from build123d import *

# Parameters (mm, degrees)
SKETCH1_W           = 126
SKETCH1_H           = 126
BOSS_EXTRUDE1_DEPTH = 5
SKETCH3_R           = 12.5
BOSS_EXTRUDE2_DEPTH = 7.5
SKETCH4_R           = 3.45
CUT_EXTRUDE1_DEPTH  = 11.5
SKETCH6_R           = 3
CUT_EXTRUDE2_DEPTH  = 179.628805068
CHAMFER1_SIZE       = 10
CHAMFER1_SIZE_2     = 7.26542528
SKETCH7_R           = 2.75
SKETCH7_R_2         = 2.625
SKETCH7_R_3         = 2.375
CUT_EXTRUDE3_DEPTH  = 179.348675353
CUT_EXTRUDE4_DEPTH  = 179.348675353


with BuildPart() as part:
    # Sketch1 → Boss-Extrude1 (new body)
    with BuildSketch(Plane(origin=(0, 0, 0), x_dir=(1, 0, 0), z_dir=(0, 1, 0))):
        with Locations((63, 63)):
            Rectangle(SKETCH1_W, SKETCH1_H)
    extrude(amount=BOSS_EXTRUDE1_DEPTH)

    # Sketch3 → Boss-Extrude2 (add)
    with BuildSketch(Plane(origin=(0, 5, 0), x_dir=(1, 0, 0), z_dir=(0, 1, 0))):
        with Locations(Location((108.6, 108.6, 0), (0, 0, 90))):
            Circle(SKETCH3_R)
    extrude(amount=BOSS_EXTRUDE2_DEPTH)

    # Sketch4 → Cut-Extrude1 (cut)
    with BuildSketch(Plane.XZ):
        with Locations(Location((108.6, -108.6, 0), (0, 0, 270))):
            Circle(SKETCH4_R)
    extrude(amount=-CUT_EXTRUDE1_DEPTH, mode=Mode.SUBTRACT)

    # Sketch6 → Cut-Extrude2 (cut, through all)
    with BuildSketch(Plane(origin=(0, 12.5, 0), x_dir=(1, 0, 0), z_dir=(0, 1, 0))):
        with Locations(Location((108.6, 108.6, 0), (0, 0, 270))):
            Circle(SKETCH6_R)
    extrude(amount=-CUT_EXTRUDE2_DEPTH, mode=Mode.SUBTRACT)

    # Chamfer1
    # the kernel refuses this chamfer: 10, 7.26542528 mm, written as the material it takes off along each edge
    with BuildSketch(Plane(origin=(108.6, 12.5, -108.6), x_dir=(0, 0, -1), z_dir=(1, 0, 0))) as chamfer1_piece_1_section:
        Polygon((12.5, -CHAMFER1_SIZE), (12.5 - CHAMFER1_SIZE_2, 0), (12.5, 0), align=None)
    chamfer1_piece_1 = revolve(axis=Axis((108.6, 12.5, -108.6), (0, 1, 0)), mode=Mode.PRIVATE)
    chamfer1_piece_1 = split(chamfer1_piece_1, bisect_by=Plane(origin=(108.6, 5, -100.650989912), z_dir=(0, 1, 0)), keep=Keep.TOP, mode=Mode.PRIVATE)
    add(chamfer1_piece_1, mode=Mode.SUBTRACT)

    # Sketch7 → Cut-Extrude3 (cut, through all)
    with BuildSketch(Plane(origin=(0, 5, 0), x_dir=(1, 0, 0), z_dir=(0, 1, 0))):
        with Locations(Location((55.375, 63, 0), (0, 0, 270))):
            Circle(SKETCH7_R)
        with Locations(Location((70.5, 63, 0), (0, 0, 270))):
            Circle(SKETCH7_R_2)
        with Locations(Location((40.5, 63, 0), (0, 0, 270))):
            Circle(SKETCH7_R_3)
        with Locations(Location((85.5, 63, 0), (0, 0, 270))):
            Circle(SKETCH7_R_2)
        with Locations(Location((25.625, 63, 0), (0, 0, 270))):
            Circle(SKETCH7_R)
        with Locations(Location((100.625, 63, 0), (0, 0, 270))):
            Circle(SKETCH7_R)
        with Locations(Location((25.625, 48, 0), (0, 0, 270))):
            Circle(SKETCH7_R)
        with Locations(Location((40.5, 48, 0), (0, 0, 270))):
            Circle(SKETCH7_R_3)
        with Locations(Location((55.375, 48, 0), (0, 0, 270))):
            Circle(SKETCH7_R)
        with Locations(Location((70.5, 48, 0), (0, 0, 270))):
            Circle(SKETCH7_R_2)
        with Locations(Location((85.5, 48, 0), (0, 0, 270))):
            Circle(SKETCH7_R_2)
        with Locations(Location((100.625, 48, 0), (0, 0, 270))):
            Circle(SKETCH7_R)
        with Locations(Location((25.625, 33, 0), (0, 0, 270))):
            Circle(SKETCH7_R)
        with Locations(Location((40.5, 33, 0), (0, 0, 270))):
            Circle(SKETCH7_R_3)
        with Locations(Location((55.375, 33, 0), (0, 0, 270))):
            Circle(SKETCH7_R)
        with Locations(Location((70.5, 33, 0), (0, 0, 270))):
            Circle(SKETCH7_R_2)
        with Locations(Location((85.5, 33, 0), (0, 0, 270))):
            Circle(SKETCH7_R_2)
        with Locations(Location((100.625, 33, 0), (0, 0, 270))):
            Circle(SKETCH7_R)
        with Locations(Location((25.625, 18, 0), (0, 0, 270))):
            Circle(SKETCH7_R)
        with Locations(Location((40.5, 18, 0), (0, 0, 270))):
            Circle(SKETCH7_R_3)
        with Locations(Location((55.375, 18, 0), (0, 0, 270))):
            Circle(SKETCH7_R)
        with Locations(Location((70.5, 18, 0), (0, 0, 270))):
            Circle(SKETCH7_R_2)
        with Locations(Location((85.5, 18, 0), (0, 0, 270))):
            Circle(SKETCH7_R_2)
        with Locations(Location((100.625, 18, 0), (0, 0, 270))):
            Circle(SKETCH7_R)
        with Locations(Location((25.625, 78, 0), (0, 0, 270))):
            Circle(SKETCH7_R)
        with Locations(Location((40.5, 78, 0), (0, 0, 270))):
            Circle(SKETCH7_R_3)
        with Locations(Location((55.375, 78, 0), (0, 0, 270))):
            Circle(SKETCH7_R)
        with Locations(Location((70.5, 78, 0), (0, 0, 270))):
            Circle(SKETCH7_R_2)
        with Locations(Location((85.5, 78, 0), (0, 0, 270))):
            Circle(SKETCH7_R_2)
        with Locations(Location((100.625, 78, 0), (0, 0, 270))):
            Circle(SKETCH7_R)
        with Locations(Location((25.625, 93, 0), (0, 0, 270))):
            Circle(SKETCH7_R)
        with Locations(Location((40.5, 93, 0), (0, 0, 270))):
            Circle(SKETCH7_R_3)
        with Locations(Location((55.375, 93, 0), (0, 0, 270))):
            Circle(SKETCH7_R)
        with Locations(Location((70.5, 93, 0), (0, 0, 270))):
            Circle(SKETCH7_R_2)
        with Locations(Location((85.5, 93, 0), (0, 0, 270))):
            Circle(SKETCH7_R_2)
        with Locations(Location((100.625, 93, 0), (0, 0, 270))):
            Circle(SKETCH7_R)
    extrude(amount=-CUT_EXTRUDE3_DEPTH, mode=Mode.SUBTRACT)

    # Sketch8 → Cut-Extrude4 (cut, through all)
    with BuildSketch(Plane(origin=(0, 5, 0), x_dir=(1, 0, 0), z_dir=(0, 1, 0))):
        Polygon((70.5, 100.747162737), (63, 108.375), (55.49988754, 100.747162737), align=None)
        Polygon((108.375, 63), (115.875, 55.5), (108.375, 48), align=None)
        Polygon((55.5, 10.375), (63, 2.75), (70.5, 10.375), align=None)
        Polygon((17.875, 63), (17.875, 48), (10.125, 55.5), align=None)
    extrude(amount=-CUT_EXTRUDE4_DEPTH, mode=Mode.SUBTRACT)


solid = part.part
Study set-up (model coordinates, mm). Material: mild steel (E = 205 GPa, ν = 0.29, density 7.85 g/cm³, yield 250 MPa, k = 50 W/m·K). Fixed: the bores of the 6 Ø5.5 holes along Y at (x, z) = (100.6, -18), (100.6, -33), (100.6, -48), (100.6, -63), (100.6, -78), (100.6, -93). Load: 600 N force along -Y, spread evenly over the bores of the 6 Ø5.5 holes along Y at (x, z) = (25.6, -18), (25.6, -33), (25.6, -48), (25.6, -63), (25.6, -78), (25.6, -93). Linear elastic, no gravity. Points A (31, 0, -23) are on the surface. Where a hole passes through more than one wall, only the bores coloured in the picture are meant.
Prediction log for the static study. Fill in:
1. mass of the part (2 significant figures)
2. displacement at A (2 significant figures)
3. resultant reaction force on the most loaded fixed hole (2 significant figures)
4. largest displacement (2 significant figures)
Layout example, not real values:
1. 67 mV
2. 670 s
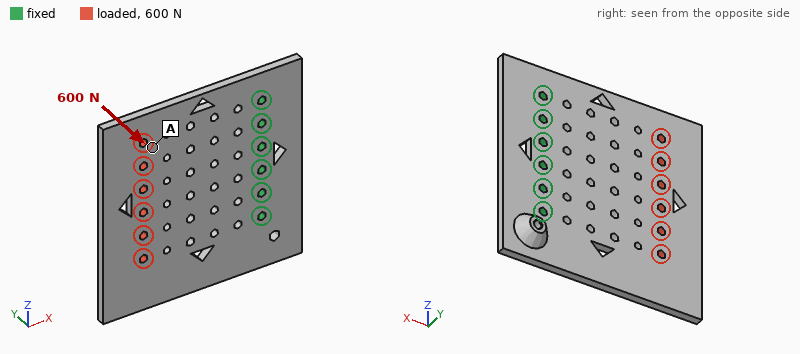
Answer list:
1. 590 g
2. 0.31 mm
3. 140 N
4. 0.54 mm
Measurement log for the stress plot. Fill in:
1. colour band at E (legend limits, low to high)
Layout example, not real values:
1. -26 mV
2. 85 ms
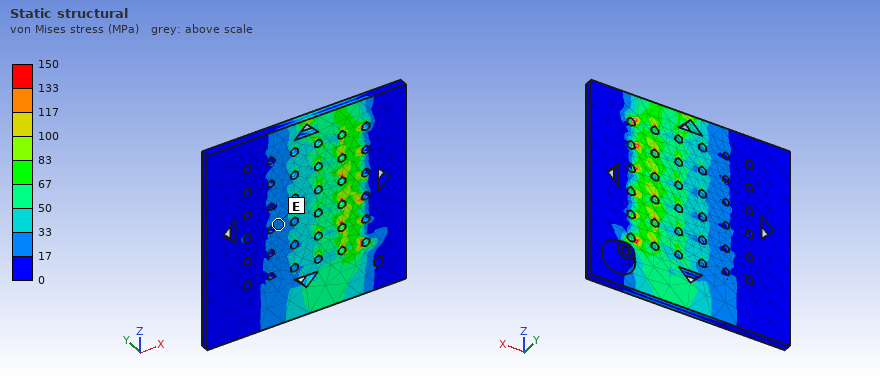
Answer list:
1. 17 to 33 MPa
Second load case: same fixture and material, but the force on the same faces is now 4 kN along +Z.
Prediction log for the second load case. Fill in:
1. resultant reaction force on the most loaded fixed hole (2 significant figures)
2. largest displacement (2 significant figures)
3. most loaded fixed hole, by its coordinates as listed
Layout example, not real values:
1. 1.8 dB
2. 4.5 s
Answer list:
1. 3.7 kN
2. 24 µm
3. (100.6, -93)
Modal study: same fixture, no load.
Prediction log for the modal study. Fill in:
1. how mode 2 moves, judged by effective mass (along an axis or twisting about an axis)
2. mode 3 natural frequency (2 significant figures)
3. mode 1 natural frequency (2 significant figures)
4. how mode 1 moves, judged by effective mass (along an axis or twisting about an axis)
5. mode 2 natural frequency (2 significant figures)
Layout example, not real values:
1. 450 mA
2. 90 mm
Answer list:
1. twisting about X
2. 2000 Hz
3. 400 Hz
4. along Y
5. 790 Hz
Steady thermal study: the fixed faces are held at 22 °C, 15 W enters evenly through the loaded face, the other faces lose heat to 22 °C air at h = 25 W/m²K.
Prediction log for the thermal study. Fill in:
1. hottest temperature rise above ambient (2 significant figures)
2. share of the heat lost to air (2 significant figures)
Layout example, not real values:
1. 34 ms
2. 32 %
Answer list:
1. 26 K
2. 60 %
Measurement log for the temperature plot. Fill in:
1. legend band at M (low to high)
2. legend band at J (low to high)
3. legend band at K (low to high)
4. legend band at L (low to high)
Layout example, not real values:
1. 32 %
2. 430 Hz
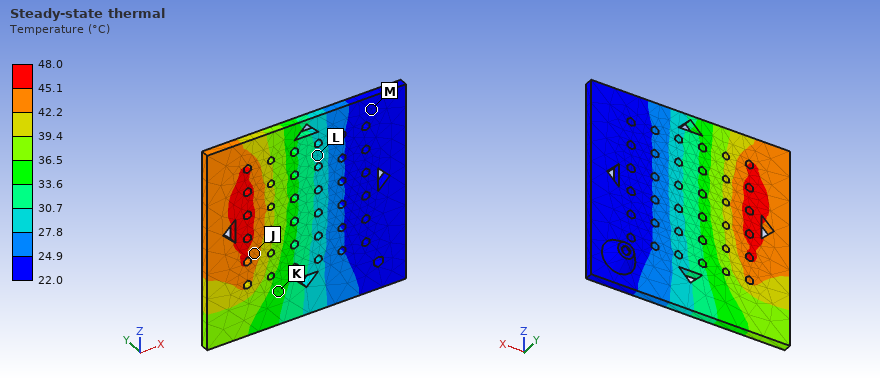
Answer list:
1. 22.0 to 24.9 °C
2. 42.2 to 45.1 °C
3. 33.6 to 36.5 °C
4. 27.8 to 30.7 °C
